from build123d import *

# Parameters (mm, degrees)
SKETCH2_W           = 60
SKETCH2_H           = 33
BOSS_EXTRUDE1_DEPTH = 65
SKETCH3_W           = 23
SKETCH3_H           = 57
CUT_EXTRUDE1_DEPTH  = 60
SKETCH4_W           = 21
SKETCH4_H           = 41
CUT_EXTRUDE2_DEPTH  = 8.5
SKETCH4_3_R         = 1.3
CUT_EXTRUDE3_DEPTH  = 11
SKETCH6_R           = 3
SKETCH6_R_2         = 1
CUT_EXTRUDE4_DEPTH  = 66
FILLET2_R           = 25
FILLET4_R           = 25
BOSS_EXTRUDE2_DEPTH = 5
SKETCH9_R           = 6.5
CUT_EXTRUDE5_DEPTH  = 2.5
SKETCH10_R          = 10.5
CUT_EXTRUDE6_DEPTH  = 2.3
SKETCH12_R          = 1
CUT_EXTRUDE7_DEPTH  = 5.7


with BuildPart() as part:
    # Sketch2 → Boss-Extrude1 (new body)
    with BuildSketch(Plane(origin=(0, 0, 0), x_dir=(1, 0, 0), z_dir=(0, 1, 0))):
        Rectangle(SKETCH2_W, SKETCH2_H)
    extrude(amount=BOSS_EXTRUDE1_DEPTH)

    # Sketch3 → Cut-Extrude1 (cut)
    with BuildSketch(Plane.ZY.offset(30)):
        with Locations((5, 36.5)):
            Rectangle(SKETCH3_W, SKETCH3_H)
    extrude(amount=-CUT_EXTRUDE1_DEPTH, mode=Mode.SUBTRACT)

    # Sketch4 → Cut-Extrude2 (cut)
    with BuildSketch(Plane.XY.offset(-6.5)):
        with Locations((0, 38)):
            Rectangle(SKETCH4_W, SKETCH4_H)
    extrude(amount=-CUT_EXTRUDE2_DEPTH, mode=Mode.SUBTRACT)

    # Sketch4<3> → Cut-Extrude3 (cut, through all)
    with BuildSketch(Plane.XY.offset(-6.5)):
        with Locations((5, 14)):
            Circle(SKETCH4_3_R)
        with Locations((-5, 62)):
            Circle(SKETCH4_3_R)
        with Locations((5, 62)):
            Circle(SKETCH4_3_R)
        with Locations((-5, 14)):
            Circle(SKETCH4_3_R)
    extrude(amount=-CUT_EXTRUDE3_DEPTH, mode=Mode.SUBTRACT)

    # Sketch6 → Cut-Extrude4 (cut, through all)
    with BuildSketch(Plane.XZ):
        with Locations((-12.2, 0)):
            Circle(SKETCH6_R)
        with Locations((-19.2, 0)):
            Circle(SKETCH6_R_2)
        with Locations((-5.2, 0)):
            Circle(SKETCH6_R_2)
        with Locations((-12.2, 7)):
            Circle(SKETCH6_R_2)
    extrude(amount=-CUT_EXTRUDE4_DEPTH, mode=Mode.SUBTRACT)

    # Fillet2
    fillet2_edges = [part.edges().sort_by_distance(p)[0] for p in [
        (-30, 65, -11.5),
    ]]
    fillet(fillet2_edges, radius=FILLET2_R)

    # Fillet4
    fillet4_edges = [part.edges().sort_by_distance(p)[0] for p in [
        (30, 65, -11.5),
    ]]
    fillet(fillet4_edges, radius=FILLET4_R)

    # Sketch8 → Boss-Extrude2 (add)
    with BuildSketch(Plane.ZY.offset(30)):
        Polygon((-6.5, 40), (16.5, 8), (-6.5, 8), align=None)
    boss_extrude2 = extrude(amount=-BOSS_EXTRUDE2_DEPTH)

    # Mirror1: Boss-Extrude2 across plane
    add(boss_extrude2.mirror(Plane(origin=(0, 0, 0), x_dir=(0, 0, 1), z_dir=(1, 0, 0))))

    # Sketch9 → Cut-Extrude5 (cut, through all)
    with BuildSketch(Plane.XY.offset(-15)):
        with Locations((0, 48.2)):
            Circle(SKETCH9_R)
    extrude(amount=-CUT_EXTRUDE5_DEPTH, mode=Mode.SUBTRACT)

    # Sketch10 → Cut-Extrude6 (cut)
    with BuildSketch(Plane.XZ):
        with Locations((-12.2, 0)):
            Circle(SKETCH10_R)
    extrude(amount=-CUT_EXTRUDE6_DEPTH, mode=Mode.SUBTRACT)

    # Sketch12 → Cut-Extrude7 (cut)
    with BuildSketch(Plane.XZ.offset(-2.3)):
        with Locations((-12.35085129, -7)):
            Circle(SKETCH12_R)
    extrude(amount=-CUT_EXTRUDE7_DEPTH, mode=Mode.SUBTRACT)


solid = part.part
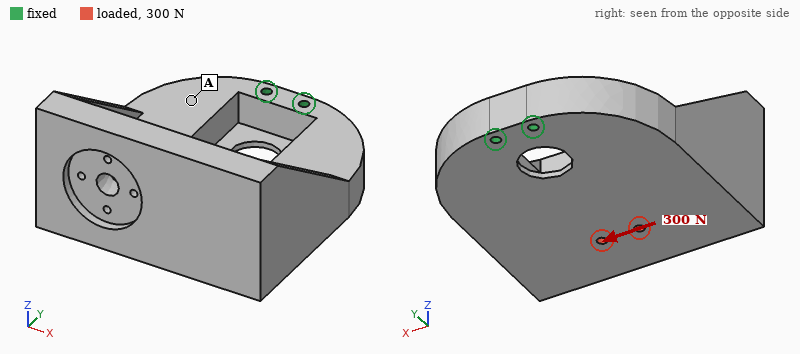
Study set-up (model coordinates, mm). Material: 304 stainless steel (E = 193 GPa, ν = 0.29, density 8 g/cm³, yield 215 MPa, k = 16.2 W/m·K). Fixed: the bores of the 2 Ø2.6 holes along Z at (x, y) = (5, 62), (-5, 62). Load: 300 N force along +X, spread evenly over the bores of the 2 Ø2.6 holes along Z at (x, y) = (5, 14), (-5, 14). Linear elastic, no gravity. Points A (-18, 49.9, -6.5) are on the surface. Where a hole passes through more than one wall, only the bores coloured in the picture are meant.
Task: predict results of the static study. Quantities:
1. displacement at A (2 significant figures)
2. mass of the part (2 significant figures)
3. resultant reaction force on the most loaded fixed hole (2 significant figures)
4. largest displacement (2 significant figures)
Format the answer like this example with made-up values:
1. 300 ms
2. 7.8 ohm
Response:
1. 8.6 µm
2. 340 g
3. 910 N
4. 32 µm
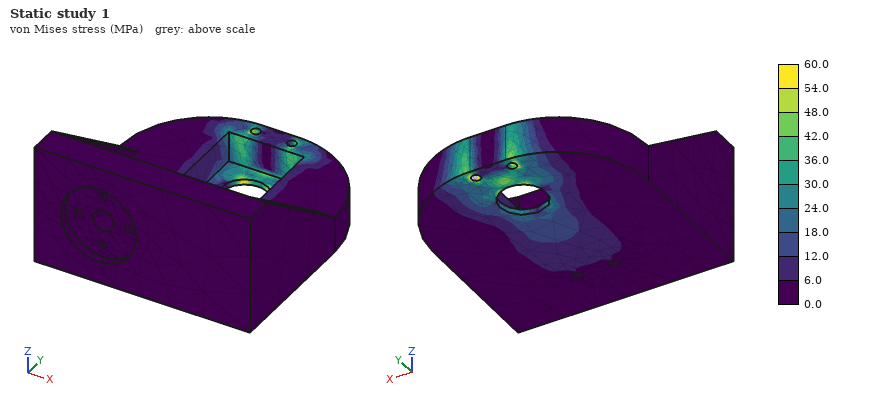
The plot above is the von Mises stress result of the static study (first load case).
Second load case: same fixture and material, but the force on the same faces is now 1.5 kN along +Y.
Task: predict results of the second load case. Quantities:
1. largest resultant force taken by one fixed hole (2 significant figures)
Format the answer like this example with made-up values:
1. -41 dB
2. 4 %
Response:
1. 790 N
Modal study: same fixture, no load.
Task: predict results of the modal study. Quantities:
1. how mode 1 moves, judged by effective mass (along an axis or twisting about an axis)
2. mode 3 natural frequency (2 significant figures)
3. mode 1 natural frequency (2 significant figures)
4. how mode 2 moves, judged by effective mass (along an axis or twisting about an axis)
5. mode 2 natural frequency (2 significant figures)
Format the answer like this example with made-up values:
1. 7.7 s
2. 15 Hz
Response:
1. along Z
2. 1900 Hz
3. 630 Hz
4. along X
5. 980 Hz
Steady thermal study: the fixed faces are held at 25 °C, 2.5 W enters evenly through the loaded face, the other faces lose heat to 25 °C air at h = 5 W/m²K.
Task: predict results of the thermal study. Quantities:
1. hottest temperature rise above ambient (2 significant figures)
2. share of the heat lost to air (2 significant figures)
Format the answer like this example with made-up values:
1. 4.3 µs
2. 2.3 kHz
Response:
1. 23 K
2. 41 %
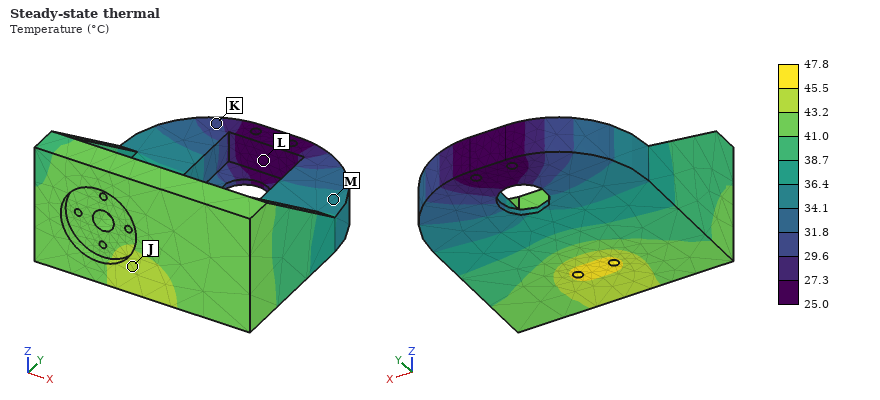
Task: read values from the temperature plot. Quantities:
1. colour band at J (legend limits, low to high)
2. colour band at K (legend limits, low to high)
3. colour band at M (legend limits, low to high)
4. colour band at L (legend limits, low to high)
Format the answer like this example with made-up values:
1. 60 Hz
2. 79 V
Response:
1. 43.2 to 45.5 °C
2. 29.6 to 31.8 °C
3. 34.1 to 36.4 °C
4. 25.0 to 27.3 °C
